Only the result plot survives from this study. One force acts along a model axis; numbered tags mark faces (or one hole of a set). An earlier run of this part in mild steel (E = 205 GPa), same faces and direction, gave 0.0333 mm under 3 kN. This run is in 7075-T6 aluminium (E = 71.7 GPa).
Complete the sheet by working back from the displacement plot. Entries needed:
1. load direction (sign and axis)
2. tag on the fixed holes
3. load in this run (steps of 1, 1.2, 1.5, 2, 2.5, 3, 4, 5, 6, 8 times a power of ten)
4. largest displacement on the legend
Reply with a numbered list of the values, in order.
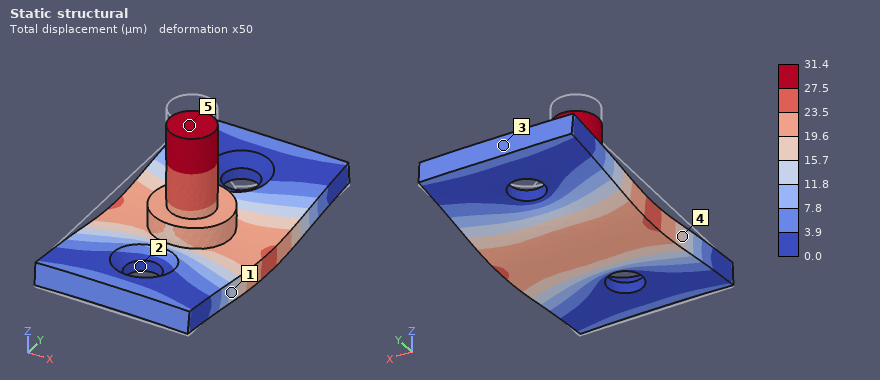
1. -Z
2. 2
3. 1 kN
4. 31.4 µm
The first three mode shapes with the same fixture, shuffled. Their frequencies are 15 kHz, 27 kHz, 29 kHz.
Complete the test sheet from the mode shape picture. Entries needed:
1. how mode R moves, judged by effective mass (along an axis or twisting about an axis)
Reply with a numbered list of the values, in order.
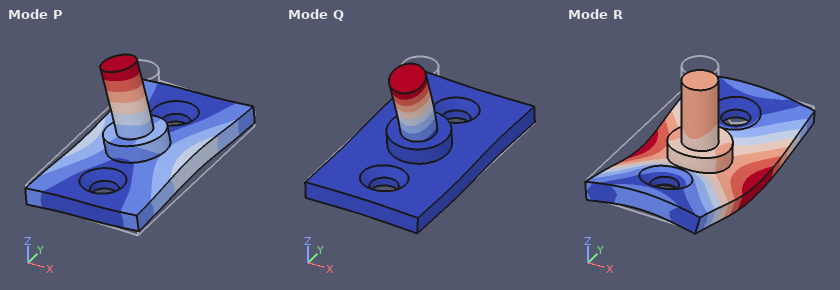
1. along Z
